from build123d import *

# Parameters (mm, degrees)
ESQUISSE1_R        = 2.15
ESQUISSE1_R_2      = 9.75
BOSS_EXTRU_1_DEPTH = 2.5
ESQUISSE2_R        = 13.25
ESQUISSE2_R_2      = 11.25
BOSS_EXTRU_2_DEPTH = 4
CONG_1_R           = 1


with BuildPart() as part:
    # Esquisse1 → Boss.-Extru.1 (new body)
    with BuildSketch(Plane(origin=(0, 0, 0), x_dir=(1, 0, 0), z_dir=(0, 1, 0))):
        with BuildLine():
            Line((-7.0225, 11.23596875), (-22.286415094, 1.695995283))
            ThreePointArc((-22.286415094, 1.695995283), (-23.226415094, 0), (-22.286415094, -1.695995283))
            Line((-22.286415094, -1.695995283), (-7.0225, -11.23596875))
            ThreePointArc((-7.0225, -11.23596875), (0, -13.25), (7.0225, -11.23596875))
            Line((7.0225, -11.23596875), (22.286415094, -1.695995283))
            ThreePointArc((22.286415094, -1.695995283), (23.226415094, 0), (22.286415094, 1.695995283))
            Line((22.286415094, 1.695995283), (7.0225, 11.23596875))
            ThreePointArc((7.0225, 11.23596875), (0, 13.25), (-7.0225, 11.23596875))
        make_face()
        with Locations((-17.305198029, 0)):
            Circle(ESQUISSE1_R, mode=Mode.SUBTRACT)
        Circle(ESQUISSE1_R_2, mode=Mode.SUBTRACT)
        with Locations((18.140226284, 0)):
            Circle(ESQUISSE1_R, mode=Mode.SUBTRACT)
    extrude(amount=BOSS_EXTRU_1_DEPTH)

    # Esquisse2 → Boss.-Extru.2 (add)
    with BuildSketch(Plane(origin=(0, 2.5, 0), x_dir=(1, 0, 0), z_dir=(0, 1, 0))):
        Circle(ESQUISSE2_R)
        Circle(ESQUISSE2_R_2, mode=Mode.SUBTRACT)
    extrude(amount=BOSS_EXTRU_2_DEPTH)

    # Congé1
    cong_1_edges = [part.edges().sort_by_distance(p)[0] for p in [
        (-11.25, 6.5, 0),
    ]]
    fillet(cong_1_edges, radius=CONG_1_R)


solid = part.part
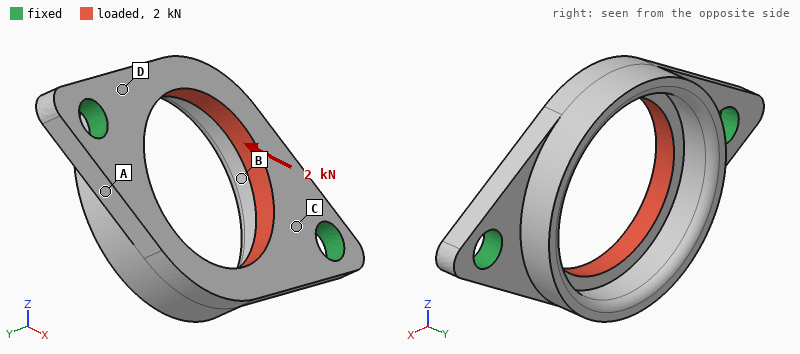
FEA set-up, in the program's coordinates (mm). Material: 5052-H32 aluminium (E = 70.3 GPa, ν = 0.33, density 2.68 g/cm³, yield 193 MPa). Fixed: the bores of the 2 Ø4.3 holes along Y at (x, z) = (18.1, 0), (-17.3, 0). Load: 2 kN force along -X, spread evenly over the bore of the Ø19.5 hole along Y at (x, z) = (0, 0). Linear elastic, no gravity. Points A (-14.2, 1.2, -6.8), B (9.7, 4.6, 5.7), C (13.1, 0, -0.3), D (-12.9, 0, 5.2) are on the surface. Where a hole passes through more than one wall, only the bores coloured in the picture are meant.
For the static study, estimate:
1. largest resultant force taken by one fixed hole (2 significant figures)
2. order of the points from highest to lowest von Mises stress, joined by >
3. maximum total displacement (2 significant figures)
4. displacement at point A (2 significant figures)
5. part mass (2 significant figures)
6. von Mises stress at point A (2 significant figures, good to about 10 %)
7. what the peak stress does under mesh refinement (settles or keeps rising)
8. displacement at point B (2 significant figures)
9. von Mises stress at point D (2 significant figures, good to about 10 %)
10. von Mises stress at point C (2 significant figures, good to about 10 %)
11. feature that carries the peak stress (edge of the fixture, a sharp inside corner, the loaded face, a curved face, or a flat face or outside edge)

1.0 kN
A > D > C > B
16 µm
5.9 µm
4.5 g
56 MPa
keeps rising
6.9 µm
42 MPa
22 MPa
edge of the fixture
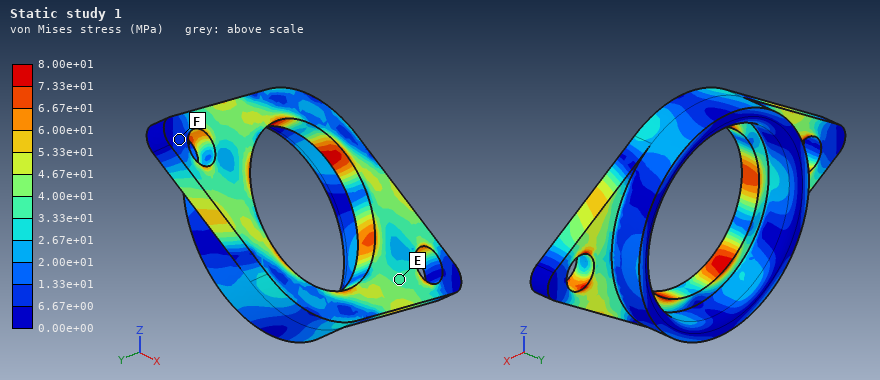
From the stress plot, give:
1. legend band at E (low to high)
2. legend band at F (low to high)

3.33e+01 to 4.00e+01 MPa
6.67e+00 to 1.33e+01 MPa
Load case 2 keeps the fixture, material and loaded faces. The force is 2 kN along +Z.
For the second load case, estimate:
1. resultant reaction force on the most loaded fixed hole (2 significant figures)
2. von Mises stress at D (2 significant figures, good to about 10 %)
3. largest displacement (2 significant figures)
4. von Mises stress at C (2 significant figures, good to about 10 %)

1.0 kN
41 MPa
20 µm
46 MPa
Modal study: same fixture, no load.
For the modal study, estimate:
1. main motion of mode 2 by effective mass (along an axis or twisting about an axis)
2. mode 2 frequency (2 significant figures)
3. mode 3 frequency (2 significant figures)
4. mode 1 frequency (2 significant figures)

along Y
11 kHz
21 kHz
8200 Hz
